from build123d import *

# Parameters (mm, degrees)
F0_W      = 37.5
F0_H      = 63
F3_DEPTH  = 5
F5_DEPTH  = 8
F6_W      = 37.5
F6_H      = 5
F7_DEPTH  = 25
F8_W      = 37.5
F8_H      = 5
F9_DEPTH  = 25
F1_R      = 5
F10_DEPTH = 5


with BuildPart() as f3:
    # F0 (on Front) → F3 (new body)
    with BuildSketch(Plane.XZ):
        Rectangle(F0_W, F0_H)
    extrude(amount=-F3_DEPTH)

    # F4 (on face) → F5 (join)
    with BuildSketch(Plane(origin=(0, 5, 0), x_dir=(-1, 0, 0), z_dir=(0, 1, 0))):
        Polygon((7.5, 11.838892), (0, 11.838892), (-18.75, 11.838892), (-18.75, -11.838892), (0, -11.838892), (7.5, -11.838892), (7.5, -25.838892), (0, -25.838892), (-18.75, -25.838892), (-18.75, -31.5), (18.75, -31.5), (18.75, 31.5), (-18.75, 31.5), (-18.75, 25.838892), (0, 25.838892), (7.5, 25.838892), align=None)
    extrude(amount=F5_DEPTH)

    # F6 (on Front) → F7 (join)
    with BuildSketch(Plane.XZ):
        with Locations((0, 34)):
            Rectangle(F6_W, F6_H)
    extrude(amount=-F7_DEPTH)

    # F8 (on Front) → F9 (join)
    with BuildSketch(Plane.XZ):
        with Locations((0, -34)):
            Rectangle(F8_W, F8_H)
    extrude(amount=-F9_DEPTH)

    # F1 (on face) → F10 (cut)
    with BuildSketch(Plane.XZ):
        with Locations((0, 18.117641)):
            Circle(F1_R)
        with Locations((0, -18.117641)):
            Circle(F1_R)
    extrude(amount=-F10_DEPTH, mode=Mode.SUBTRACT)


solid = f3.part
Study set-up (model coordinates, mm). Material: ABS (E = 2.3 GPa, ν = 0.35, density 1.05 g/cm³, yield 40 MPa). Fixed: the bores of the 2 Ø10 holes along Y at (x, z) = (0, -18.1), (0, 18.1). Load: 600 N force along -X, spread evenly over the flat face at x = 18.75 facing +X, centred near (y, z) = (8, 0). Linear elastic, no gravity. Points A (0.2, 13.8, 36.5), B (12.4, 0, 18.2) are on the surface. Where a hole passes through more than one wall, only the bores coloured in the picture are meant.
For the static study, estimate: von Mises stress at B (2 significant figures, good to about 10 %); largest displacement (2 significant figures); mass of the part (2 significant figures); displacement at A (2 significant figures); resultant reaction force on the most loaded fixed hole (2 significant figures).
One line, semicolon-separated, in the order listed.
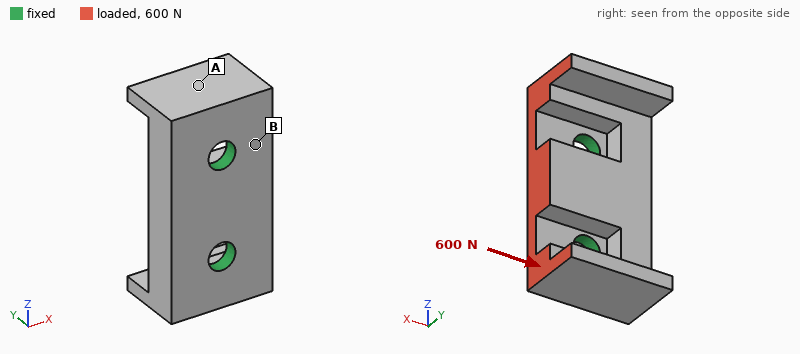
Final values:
2.2 MPa; 0.12 mm; 35 g; 0.052 mm; 300 N
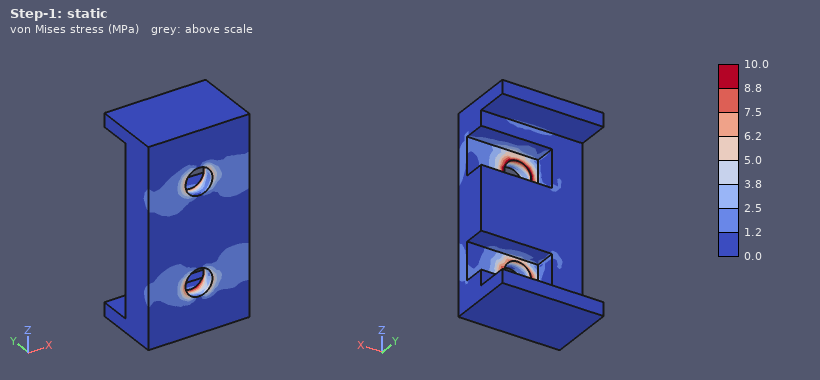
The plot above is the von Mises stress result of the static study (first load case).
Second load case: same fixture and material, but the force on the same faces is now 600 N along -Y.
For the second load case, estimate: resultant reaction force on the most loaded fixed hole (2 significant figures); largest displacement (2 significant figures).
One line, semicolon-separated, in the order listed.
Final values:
300 N; 0.45 mm
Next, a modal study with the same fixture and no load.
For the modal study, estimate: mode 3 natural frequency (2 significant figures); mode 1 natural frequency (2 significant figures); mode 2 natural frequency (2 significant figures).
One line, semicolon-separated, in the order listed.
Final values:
2200 Hz; 2000 Hz; 2100 Hz
